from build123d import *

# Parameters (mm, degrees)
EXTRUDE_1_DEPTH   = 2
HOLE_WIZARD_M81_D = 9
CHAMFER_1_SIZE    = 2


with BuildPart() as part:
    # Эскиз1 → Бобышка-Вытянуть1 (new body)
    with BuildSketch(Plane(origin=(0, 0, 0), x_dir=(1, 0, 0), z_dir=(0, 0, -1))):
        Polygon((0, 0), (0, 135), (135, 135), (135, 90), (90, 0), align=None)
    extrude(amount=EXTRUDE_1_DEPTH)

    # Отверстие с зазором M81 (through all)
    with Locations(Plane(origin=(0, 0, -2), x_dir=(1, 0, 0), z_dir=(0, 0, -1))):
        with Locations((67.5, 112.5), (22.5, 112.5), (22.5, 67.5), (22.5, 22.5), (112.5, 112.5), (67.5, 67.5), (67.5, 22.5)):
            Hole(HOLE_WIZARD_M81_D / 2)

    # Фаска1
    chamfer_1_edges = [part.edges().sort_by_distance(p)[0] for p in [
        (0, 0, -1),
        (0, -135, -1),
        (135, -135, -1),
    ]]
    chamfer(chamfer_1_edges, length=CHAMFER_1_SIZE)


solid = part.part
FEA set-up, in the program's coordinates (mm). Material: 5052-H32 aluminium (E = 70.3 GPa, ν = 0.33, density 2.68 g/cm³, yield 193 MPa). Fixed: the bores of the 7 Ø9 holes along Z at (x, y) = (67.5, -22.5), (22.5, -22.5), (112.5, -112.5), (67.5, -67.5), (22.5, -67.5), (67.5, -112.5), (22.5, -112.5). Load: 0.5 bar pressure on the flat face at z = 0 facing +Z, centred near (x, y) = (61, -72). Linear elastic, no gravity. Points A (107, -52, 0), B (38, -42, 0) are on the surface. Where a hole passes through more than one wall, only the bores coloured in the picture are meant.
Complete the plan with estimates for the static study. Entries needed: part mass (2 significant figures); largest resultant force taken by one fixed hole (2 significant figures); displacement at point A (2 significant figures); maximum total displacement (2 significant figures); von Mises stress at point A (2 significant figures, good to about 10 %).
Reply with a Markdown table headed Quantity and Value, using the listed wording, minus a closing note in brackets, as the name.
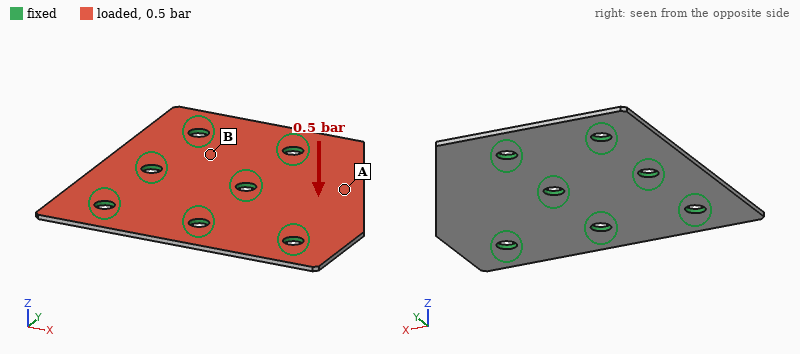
| Quantity | Value |
|---|---|
| part mass | 84 g |
| largest resultant force taken by one fixed hole | 140 N |
| displacement at point A | 0.23 mm |
| maximum total displacement | 0.30 mm |
| von Mises stress at point A | 13 MPa |
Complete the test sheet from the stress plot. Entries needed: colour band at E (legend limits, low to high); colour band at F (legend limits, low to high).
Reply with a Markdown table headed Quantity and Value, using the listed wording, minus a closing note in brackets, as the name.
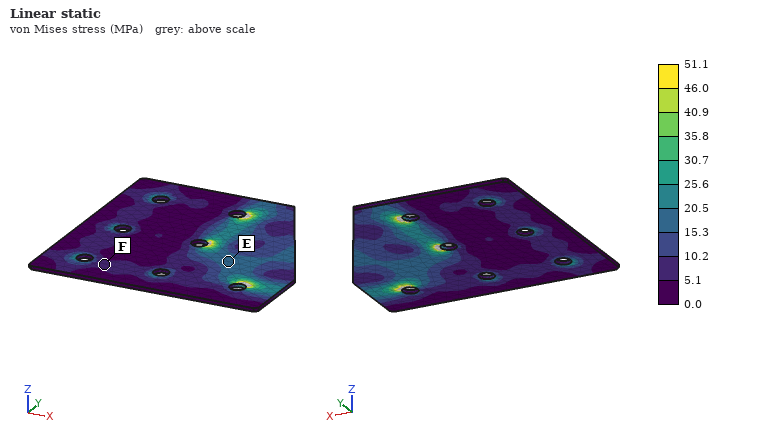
| Quantity | Value |
|---|---|
| colour band at E | 15.3 to 20.5 MPa |
| colour band at F | 5.1 to 10.2 MPa |
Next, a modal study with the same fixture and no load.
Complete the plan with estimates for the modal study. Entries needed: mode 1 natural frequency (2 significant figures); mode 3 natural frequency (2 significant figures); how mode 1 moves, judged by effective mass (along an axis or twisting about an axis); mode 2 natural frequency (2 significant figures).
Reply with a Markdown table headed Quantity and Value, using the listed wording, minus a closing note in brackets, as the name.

| Quantity | Value |
|---|---|
| mode 1 natural frequency | 1200 Hz |
| mode 3 natural frequency | 3100 Hz |
| how mode 1 moves, judged by effective mass | along Z |
| mode 2 natural frequency | 2300 Hz |
